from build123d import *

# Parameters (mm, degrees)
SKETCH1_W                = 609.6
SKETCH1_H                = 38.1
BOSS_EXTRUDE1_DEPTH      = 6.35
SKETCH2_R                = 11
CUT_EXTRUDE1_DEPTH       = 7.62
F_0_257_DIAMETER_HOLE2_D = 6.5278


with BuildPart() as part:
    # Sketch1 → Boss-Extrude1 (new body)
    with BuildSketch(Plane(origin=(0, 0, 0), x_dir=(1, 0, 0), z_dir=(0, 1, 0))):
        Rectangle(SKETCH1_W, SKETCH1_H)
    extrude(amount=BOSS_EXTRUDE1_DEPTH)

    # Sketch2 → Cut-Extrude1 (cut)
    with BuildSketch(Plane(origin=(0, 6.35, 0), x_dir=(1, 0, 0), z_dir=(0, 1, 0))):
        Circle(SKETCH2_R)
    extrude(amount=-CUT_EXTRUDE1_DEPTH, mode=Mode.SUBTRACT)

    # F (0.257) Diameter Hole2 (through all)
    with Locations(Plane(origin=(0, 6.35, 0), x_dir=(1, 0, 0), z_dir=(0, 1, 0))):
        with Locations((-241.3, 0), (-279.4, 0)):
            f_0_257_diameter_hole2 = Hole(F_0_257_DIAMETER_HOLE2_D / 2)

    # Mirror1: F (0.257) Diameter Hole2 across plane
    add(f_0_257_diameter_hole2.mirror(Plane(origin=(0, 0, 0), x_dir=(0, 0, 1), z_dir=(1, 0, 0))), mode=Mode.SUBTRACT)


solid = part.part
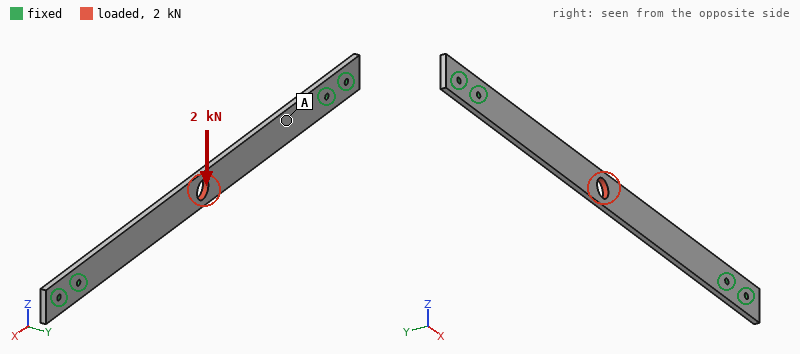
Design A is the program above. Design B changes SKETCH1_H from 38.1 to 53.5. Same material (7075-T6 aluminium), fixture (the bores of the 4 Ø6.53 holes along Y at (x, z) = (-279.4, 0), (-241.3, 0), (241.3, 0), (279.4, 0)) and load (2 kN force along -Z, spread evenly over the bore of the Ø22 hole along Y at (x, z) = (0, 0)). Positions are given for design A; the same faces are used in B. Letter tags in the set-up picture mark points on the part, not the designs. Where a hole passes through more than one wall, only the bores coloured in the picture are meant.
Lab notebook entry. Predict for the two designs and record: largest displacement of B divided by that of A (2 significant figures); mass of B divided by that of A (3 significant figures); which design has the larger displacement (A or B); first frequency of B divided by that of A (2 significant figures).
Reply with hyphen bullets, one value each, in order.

- 0.41
- 1.41
- A
- 1.00
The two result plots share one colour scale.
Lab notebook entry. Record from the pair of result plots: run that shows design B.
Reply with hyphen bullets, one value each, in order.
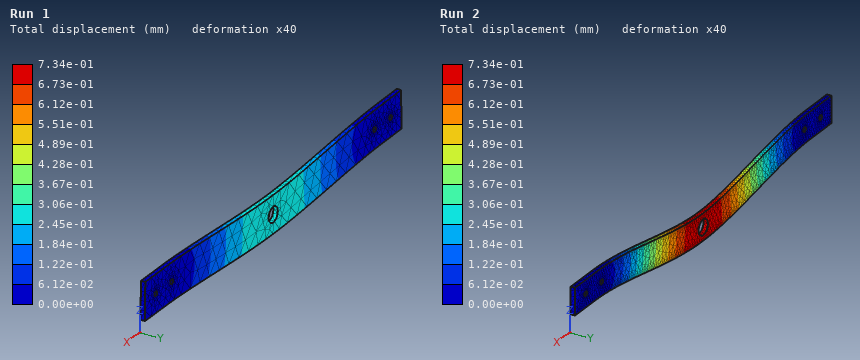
- Run 1
